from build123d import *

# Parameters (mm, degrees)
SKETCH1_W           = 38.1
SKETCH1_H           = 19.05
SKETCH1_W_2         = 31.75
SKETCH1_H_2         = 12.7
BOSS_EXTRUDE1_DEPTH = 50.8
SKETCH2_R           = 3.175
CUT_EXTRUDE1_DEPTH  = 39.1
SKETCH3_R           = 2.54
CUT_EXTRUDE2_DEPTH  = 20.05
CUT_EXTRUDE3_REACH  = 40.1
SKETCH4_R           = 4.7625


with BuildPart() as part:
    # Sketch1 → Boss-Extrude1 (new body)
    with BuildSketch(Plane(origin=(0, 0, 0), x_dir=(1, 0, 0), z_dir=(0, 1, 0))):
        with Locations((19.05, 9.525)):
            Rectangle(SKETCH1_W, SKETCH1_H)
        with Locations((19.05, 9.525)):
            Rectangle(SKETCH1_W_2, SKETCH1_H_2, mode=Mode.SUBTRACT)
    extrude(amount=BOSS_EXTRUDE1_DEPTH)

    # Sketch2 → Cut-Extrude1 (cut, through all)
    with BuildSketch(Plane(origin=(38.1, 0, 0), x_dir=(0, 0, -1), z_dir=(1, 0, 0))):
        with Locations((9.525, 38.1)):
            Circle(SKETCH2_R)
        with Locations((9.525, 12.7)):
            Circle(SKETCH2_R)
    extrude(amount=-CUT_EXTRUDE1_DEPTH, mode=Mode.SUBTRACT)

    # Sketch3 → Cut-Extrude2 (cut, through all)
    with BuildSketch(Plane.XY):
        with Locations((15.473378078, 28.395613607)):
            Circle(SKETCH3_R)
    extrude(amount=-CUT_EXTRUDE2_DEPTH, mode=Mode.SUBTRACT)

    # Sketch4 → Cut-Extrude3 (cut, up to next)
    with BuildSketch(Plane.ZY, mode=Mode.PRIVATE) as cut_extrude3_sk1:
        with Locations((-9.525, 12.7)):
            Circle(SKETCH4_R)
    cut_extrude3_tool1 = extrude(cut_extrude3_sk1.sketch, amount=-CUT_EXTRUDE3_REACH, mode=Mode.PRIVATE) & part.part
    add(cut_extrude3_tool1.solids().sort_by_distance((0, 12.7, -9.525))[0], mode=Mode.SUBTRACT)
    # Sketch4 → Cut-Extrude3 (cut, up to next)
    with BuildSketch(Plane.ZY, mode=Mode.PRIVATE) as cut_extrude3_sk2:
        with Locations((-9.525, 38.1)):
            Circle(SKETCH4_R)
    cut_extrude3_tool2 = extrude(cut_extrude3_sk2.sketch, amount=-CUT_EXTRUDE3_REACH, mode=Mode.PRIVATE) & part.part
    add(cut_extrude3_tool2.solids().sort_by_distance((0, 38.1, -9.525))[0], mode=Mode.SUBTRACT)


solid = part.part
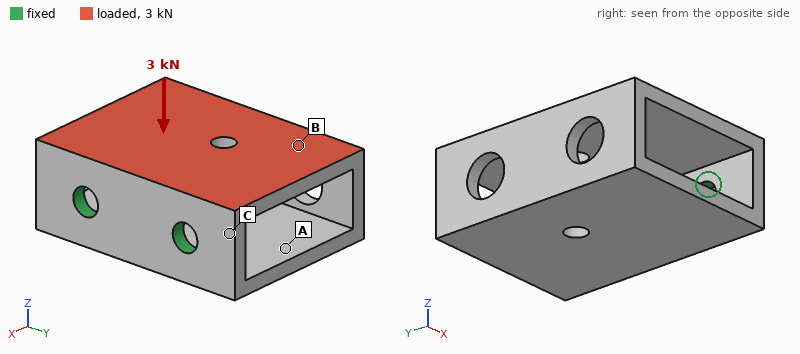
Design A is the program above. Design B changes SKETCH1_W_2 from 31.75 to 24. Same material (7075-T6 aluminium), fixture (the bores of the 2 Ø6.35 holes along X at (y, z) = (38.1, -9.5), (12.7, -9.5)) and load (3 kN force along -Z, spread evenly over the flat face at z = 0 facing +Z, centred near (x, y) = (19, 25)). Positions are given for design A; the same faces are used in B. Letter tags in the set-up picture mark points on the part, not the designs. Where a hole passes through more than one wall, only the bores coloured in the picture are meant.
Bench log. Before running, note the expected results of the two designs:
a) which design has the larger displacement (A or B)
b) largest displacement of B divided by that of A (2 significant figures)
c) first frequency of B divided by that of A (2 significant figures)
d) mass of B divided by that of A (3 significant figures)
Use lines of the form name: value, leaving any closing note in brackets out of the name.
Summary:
which design has the larger displacement: A
largest displacement of B divided by that of A: 0.27
first frequency of B divided by that of A: 1.7
mass of B divided by that of A: 1.27
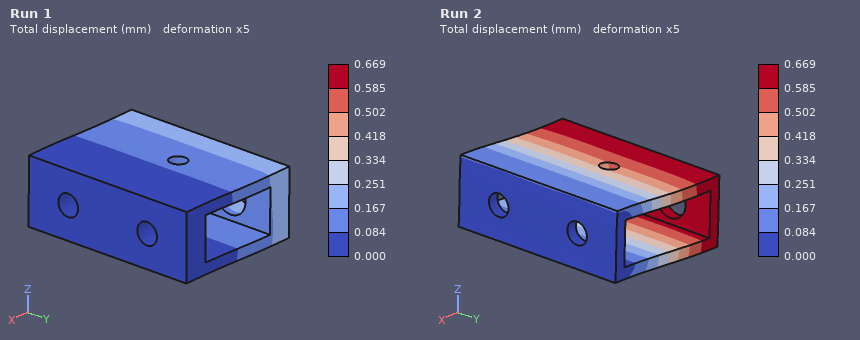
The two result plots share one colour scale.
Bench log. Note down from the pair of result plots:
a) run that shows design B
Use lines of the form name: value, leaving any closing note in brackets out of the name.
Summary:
run that shows design B: Run 1
